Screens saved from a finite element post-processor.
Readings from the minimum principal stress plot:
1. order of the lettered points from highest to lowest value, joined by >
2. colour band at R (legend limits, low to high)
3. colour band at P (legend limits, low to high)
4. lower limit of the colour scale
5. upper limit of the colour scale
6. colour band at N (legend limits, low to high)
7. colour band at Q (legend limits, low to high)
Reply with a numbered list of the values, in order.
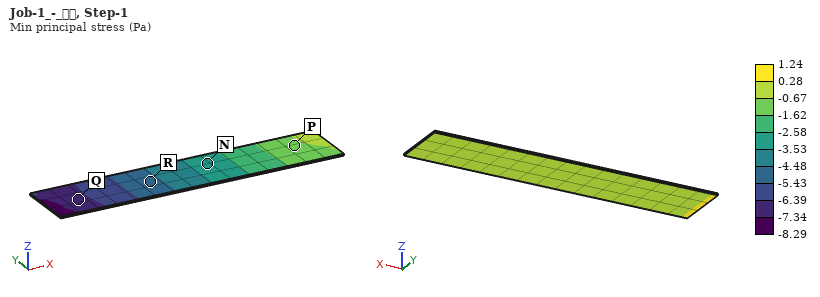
1. P > N > R > Q
2. -5.43 to -4.48 Pa
3. -1.62 to -0.67 Pa
4. -8.29 Pa
5. 1.24 Pa
6. -3.53 to -2.58 Pa
7. -7.34 to -6.39 Pa
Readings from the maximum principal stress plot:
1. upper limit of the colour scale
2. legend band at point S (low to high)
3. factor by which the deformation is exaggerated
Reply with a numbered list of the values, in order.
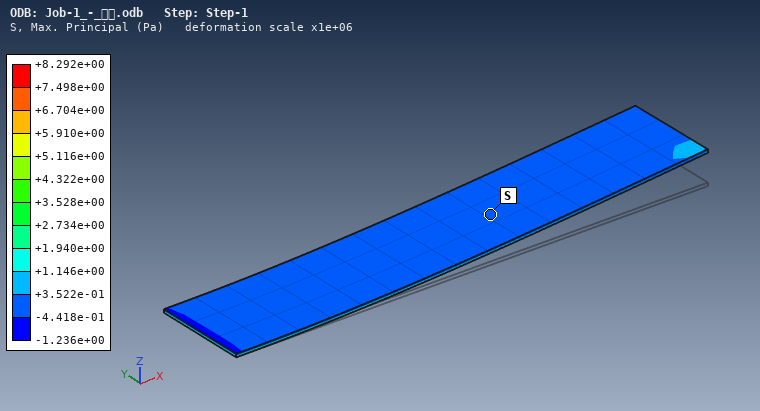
1. +8.292e+00 Pa
2. -4.418e-01 to +3.522e-01 Pa
3. 1e+06
